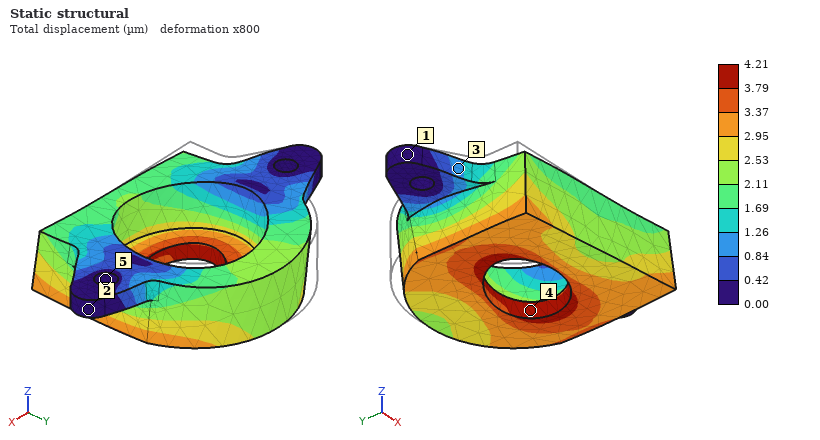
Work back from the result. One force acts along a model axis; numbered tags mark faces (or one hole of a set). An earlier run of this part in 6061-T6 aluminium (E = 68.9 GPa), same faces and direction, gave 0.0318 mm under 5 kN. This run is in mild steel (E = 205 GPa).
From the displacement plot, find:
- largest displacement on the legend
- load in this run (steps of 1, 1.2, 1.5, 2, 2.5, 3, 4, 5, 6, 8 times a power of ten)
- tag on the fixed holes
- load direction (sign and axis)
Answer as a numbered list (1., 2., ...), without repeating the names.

1. 4.21 µm
2. 2 kN
3. 5
4. +X
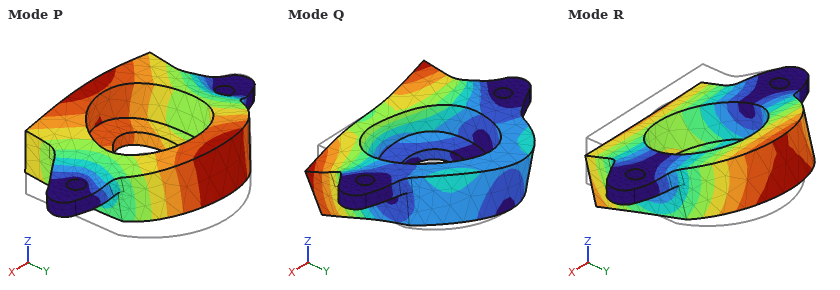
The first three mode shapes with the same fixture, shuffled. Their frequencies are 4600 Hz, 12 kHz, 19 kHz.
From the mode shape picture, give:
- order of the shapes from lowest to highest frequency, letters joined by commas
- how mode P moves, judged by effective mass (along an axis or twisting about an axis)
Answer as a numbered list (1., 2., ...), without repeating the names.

1. R, P, Q
2. along Z
